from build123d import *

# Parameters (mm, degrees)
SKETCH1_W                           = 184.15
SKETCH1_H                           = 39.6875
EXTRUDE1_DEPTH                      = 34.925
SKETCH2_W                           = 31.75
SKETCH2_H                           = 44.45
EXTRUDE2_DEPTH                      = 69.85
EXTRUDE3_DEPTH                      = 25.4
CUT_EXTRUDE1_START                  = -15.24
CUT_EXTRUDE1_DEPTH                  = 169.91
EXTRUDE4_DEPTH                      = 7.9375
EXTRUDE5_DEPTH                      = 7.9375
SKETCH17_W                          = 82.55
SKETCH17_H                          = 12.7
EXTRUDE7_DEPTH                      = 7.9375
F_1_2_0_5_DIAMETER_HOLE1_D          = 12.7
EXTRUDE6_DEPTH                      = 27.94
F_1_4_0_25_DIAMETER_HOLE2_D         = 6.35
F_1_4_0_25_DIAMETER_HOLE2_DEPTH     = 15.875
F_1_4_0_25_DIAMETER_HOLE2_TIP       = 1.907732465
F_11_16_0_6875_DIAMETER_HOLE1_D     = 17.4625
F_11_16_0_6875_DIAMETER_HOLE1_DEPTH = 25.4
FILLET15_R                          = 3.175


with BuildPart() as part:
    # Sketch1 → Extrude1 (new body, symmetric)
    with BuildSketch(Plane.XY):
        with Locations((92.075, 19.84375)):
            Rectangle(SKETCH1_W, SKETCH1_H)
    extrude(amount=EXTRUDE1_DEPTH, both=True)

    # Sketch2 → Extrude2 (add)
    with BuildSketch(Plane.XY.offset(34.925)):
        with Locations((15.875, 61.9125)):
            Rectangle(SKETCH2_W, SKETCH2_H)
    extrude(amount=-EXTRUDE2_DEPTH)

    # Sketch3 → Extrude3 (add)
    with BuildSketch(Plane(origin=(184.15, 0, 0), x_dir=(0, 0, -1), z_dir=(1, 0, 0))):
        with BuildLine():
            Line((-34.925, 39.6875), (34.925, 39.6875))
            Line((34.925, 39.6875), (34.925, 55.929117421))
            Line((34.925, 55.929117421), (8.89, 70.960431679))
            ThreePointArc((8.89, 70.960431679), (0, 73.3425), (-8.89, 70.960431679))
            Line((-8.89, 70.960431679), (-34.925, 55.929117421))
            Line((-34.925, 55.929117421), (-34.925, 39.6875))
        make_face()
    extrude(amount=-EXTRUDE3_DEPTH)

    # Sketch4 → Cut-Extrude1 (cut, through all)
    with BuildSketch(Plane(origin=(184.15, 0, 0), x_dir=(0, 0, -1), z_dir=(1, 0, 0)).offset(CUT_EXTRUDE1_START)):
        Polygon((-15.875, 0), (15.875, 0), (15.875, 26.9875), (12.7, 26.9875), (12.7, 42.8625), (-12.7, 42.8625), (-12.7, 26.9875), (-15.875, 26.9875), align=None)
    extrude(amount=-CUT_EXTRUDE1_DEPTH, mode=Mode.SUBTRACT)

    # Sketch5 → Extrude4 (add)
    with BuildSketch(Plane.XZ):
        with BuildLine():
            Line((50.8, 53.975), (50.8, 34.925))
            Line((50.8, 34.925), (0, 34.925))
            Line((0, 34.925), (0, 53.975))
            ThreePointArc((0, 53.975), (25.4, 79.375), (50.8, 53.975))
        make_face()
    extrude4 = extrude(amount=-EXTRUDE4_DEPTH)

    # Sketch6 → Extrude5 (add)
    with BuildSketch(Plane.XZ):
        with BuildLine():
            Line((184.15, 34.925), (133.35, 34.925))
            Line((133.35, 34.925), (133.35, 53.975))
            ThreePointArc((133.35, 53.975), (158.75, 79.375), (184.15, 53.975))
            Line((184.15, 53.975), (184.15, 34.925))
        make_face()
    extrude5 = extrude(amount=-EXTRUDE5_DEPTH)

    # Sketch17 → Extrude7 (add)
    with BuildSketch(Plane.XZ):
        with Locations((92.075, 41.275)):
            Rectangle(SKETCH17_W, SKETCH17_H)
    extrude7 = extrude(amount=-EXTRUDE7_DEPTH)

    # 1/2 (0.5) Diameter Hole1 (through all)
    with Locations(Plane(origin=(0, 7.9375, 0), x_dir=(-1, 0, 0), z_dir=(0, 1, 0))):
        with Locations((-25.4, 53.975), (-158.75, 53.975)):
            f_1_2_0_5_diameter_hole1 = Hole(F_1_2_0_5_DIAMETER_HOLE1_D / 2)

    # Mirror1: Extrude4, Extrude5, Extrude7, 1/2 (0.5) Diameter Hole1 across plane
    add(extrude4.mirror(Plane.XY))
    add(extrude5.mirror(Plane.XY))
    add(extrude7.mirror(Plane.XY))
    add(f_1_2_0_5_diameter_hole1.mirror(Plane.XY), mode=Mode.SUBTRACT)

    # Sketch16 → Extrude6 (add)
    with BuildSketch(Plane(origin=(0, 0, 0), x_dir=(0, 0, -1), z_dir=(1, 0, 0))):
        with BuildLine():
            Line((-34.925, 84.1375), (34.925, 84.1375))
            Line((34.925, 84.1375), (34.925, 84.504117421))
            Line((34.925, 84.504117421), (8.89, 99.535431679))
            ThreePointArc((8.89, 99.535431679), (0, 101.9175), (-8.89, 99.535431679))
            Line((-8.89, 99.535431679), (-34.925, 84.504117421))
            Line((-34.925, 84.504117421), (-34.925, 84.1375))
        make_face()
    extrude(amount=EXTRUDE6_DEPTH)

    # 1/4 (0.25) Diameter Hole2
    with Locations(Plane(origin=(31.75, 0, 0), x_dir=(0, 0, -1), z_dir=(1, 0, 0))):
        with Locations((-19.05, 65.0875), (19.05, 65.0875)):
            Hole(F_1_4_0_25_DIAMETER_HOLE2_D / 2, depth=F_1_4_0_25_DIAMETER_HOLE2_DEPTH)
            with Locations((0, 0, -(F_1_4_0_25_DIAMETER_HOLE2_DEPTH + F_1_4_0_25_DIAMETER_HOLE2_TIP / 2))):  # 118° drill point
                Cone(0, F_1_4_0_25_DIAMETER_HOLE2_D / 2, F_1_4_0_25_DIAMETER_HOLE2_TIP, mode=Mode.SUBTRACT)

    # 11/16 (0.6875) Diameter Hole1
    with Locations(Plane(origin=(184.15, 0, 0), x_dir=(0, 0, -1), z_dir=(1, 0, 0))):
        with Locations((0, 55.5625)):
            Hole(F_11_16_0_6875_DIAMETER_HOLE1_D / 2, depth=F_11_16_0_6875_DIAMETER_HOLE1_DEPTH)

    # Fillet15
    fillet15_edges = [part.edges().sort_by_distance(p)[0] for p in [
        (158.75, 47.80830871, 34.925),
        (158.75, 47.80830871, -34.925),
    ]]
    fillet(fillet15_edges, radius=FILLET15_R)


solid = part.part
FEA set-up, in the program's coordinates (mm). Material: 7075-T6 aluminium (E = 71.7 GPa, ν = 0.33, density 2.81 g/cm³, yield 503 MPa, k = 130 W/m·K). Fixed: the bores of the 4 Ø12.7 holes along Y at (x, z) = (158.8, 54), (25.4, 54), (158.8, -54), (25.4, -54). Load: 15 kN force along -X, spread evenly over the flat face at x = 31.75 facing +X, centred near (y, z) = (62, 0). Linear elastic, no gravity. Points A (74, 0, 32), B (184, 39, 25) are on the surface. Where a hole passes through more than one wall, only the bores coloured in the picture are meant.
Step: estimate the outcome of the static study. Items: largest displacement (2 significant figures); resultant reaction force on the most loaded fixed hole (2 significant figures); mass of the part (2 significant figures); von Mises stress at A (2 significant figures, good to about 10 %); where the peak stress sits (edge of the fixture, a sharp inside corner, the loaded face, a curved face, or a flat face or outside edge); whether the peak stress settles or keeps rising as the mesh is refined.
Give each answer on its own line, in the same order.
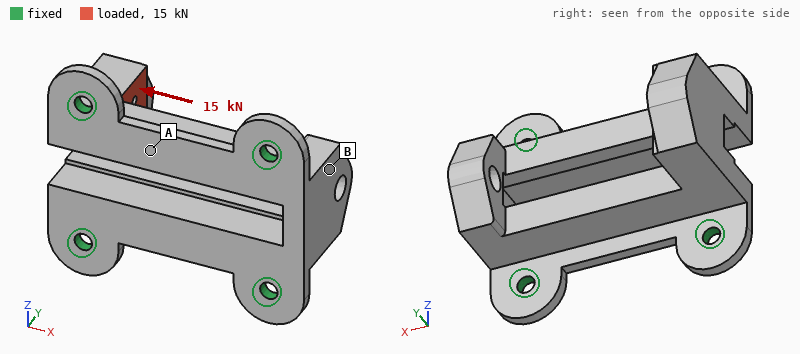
0.28 mm
6.3 kN
1.5 kg
21 MPa
edge of the fixture
keeps rising
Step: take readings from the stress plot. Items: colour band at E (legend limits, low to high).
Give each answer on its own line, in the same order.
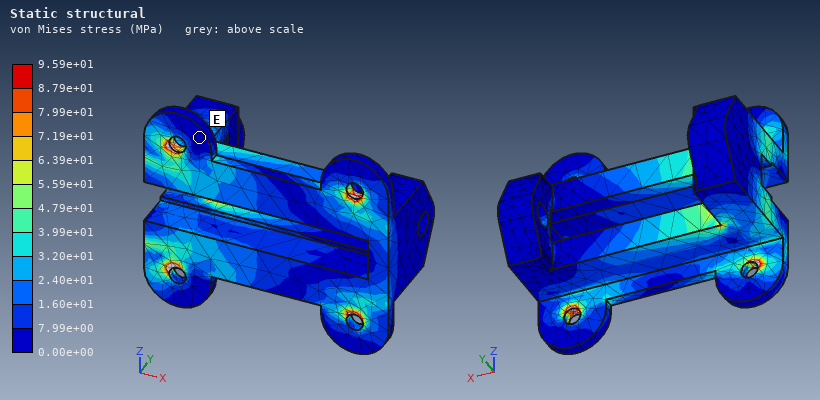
0.00e+00 to 7.99e+00 MPa
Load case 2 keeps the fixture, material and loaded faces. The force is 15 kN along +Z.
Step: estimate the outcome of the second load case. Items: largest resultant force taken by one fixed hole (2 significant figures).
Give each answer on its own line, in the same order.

12 kN
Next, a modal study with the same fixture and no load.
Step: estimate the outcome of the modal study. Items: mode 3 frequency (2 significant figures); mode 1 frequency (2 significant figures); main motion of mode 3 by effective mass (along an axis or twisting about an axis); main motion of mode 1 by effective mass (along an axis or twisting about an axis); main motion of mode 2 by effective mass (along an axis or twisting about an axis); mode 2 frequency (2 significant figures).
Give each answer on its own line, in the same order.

2700 Hz
2100 Hz
along Y
along X
along Z
2400 Hz
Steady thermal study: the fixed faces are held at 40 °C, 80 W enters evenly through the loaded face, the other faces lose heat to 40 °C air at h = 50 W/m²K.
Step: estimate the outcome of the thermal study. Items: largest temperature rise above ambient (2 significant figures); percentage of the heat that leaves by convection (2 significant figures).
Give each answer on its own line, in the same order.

26 K
38 %
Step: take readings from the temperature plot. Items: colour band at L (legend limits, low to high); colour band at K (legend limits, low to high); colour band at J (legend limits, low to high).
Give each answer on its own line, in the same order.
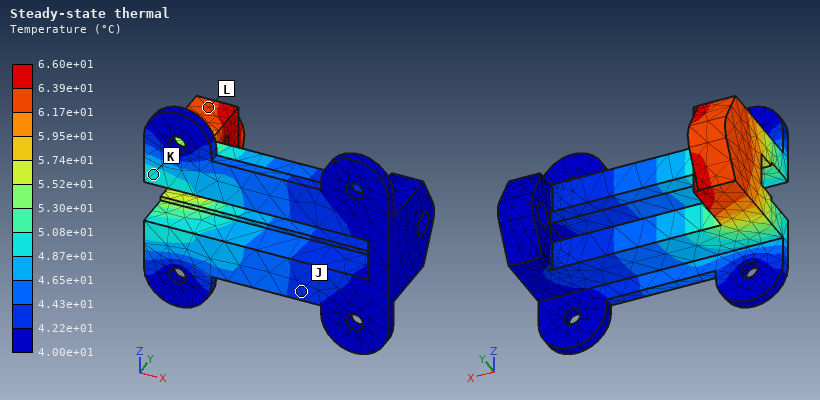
6.17e+01 to 6.39e+01 °C
4.87e+01 to 5.08e+01 °C
4.22e+01 to 4.43e+01 °C
